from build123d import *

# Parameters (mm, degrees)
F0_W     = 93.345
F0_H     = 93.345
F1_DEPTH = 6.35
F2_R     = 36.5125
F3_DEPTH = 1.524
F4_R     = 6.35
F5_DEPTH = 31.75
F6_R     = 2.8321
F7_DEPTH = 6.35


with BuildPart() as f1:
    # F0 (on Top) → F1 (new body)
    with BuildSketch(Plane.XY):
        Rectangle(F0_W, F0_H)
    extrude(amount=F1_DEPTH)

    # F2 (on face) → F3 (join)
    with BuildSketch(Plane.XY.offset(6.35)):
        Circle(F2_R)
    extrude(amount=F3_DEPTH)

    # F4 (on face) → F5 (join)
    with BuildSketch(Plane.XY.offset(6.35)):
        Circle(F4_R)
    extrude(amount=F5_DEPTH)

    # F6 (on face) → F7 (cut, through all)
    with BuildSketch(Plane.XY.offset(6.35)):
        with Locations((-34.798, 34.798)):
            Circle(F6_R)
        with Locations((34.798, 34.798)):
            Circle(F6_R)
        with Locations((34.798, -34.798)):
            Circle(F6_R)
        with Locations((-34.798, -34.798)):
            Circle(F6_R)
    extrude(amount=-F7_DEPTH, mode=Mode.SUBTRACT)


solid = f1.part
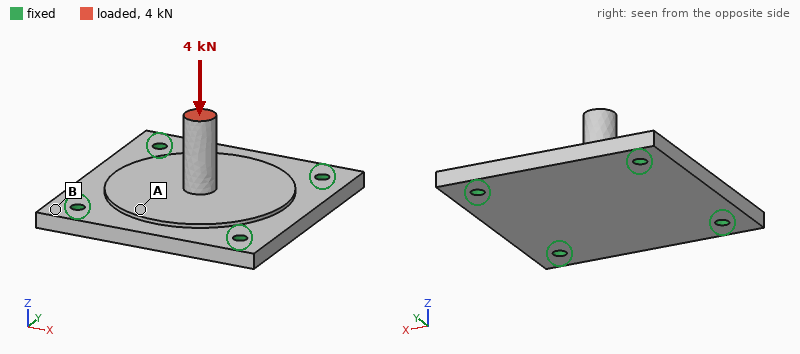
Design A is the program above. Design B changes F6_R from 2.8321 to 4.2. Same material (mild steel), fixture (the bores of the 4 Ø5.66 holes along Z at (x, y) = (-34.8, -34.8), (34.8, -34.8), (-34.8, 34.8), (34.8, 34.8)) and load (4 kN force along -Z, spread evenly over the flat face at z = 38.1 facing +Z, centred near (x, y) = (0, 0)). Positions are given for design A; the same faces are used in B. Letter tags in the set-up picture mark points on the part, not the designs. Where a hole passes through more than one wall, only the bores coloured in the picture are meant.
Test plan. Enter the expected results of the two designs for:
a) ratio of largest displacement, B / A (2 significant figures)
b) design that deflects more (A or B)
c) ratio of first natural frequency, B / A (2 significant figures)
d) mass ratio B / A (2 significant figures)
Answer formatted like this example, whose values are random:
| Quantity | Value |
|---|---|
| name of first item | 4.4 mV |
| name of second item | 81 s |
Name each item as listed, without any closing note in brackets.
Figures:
| Quantity | Value |
|---|---|
| ratio of largest displacement, B / A | 0.91 |
| design that deflects more | A |
| ratio of first natural frequency, B / A | 1.1 |
| mass ratio B / A | 0.99 |
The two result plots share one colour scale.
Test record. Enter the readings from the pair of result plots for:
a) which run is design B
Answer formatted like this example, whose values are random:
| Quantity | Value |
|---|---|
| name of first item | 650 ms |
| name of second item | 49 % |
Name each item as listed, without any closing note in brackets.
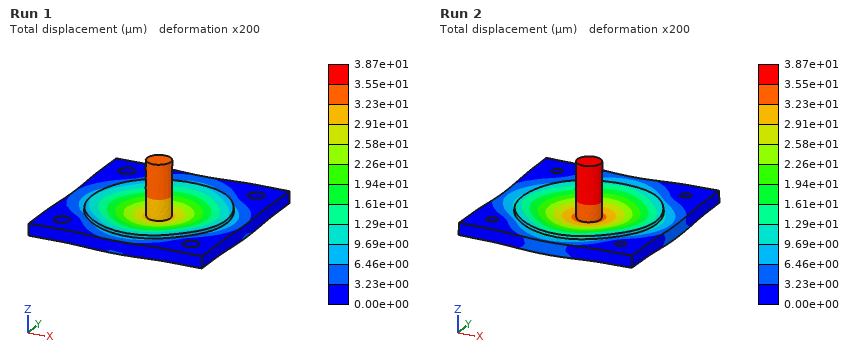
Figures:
| Quantity | Value |
|---|---|
| which run is design B | Run 1 |
